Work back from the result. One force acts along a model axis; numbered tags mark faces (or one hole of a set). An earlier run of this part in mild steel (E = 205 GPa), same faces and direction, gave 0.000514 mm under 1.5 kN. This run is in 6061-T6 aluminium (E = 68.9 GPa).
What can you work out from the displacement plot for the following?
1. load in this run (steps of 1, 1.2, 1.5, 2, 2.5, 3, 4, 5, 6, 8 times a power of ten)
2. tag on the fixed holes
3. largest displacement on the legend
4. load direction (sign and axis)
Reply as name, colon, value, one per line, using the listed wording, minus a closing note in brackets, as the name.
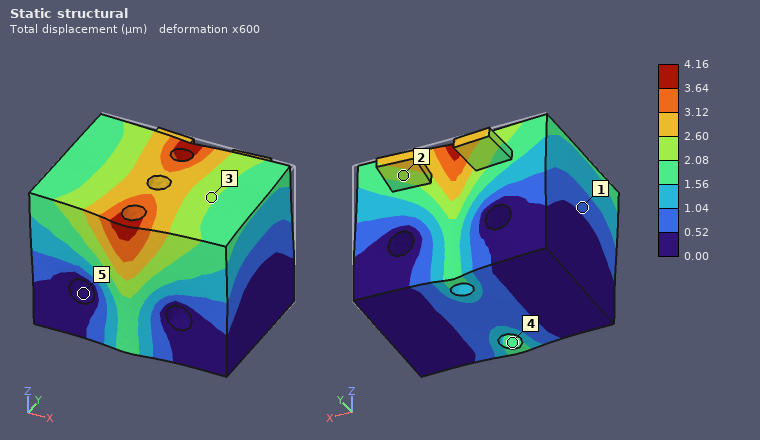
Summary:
load in this run: 4 kN
tag on the fixed holes: 5
largest displacement on the legend: 4.16 µm
load direction: -Y
